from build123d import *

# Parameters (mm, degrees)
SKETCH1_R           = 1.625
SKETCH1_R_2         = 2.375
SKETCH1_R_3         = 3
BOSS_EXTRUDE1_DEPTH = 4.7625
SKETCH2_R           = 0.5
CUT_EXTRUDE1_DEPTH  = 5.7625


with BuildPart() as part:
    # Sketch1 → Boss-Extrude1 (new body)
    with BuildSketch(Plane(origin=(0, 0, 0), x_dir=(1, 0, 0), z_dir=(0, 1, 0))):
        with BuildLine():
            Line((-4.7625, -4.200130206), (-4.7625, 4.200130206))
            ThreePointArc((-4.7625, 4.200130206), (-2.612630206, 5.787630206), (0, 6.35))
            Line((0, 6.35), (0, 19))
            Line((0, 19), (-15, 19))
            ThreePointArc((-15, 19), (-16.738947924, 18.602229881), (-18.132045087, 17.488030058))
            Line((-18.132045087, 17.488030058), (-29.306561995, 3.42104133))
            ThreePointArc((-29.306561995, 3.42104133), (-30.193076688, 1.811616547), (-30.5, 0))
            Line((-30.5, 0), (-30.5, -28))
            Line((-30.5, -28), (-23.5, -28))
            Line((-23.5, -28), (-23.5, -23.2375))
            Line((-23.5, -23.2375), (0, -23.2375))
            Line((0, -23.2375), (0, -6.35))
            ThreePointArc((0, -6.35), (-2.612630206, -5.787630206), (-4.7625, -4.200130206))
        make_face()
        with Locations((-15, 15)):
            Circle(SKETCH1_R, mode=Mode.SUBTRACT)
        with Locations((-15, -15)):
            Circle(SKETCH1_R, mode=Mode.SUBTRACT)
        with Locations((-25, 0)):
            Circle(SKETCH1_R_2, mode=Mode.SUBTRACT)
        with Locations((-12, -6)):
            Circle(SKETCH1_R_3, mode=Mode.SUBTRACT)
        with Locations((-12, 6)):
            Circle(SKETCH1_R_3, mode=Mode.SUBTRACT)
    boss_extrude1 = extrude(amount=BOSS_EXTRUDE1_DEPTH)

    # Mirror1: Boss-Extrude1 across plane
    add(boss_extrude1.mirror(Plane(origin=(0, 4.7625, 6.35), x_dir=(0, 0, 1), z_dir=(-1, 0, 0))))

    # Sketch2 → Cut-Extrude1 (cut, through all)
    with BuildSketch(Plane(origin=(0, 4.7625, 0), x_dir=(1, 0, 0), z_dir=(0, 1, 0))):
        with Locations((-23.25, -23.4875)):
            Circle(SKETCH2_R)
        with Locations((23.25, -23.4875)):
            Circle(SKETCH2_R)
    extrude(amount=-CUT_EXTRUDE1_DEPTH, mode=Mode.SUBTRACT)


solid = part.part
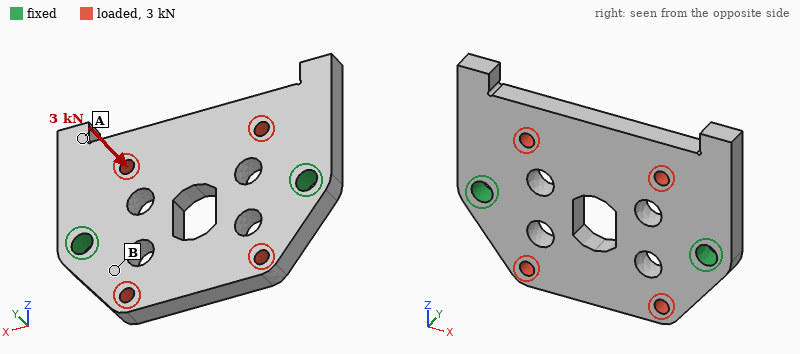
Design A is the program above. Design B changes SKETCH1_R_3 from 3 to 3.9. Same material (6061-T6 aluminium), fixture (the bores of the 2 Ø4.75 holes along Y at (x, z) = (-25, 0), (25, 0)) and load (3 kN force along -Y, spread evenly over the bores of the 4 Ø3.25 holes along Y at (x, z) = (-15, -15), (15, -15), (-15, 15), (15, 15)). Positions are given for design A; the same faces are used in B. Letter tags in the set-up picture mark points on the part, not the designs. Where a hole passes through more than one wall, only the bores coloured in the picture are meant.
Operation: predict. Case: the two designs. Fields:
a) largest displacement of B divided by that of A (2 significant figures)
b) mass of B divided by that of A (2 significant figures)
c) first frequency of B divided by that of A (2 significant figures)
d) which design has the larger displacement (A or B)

1.1
0.96
0.98
B
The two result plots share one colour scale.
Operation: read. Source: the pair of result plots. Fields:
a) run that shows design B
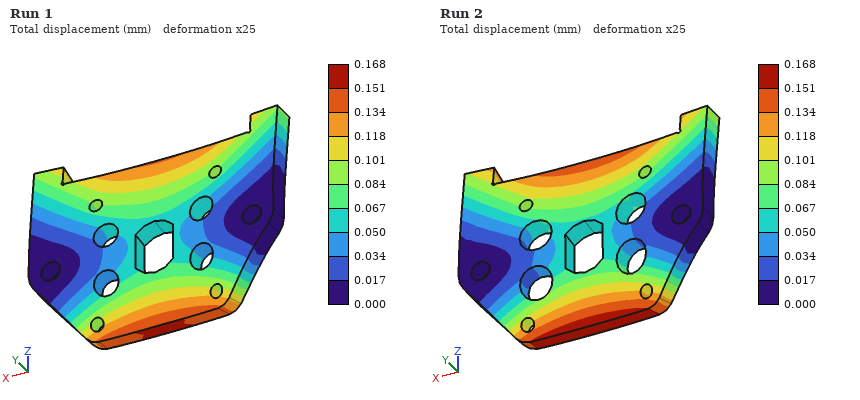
Run 2
